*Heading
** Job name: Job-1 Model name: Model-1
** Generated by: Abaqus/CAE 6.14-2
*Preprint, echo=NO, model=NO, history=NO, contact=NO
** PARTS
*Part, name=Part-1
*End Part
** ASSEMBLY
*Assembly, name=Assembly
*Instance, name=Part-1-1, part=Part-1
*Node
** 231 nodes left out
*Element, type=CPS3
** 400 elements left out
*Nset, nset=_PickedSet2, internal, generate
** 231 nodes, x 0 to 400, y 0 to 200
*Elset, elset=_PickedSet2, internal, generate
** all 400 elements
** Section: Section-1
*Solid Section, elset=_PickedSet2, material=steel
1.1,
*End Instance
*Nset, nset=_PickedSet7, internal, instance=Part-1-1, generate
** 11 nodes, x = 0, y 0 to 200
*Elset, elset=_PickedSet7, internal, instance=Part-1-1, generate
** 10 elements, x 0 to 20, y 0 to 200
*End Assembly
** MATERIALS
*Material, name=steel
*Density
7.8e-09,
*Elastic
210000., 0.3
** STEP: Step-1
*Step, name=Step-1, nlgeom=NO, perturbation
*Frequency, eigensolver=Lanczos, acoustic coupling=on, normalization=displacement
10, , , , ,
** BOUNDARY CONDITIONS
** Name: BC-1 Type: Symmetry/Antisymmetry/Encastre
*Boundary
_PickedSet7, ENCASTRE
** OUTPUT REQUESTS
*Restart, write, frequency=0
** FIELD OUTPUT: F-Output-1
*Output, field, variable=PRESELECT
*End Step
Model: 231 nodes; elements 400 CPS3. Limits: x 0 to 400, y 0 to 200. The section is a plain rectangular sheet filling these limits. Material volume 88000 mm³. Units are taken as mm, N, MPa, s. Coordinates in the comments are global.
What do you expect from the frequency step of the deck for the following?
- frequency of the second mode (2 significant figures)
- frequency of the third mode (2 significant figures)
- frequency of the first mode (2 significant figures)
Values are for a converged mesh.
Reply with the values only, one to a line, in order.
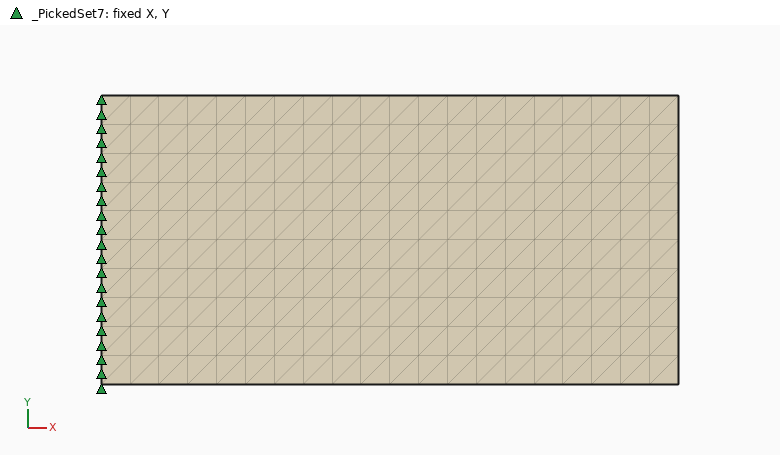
3300 Hz
3400 Hz
900 Hz
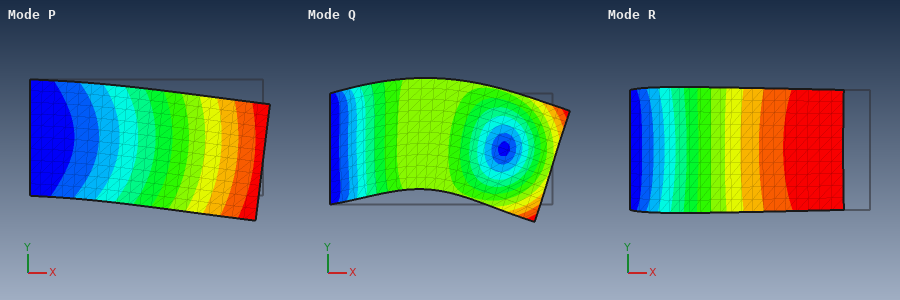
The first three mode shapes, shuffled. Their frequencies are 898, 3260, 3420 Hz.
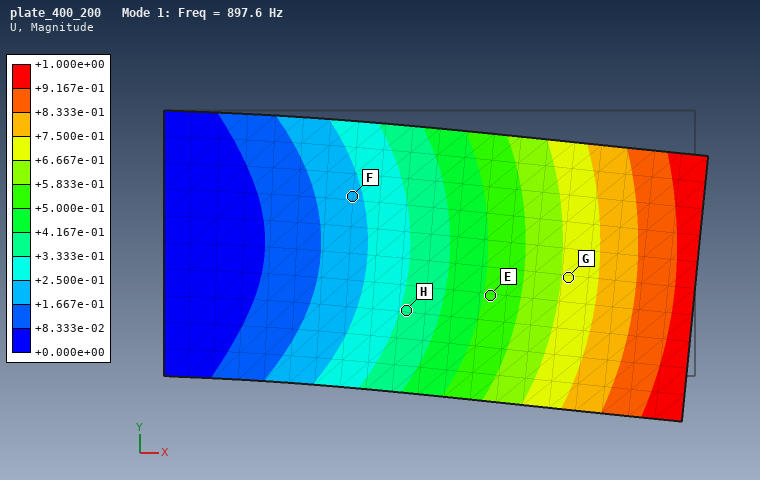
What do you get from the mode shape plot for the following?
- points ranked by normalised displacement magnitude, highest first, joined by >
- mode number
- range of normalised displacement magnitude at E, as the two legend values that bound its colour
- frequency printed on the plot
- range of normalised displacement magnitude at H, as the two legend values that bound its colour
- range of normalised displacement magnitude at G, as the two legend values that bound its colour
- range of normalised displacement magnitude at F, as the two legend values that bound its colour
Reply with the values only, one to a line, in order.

G > E > H > F
1
+5.000e-01 to +5.833e-01
897.6 Hz
+3.333e-01 to +4.167e-01
+6.667e-01 to +7.500e-01
+1.667e-01 to +2.500e-01
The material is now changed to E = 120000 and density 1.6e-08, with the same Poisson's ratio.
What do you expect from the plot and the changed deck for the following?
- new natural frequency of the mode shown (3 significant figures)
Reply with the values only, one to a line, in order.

474 Hz
